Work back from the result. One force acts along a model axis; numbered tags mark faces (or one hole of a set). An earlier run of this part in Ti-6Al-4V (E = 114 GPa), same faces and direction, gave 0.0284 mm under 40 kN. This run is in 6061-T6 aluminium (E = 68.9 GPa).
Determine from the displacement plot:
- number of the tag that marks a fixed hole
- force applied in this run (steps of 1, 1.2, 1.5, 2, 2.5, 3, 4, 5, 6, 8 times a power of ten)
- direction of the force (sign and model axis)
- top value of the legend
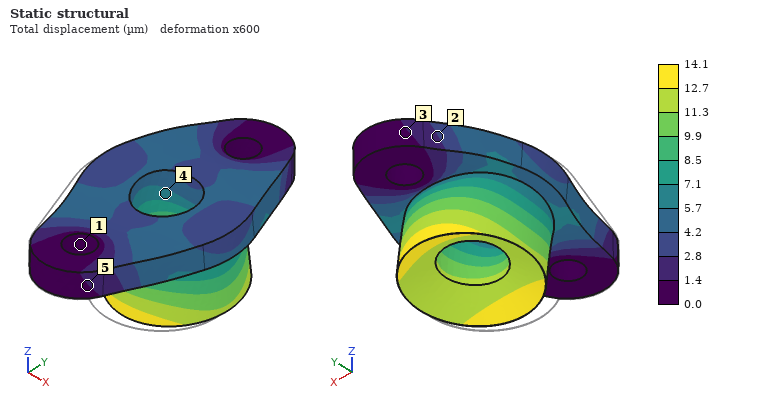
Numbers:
1
12 kN
+Y
14.1 µm
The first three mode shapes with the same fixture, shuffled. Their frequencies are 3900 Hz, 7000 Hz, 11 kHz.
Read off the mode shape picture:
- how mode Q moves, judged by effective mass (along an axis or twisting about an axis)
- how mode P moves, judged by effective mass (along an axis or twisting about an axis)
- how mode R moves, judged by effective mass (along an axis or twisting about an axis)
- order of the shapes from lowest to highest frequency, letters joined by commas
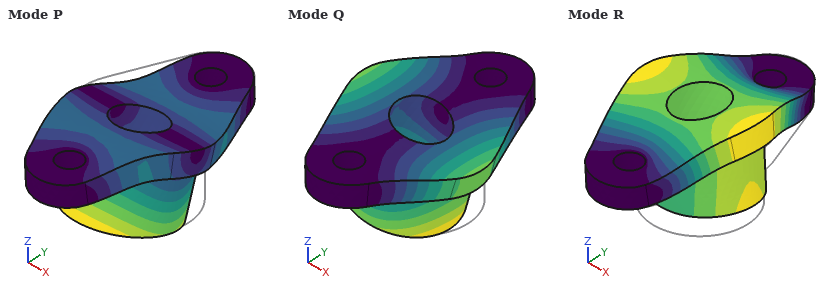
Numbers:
along X
along Y
along Z
Q, R, P
